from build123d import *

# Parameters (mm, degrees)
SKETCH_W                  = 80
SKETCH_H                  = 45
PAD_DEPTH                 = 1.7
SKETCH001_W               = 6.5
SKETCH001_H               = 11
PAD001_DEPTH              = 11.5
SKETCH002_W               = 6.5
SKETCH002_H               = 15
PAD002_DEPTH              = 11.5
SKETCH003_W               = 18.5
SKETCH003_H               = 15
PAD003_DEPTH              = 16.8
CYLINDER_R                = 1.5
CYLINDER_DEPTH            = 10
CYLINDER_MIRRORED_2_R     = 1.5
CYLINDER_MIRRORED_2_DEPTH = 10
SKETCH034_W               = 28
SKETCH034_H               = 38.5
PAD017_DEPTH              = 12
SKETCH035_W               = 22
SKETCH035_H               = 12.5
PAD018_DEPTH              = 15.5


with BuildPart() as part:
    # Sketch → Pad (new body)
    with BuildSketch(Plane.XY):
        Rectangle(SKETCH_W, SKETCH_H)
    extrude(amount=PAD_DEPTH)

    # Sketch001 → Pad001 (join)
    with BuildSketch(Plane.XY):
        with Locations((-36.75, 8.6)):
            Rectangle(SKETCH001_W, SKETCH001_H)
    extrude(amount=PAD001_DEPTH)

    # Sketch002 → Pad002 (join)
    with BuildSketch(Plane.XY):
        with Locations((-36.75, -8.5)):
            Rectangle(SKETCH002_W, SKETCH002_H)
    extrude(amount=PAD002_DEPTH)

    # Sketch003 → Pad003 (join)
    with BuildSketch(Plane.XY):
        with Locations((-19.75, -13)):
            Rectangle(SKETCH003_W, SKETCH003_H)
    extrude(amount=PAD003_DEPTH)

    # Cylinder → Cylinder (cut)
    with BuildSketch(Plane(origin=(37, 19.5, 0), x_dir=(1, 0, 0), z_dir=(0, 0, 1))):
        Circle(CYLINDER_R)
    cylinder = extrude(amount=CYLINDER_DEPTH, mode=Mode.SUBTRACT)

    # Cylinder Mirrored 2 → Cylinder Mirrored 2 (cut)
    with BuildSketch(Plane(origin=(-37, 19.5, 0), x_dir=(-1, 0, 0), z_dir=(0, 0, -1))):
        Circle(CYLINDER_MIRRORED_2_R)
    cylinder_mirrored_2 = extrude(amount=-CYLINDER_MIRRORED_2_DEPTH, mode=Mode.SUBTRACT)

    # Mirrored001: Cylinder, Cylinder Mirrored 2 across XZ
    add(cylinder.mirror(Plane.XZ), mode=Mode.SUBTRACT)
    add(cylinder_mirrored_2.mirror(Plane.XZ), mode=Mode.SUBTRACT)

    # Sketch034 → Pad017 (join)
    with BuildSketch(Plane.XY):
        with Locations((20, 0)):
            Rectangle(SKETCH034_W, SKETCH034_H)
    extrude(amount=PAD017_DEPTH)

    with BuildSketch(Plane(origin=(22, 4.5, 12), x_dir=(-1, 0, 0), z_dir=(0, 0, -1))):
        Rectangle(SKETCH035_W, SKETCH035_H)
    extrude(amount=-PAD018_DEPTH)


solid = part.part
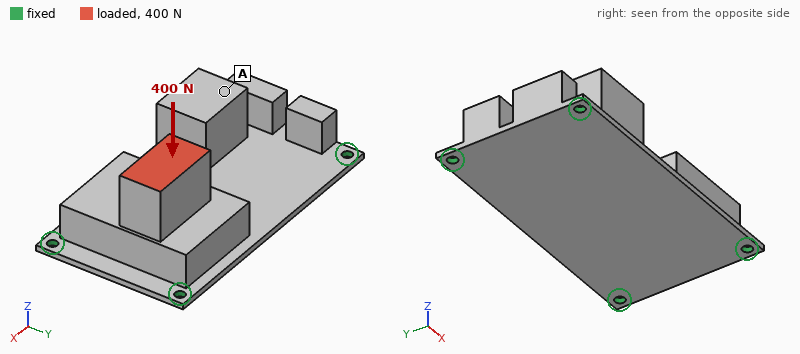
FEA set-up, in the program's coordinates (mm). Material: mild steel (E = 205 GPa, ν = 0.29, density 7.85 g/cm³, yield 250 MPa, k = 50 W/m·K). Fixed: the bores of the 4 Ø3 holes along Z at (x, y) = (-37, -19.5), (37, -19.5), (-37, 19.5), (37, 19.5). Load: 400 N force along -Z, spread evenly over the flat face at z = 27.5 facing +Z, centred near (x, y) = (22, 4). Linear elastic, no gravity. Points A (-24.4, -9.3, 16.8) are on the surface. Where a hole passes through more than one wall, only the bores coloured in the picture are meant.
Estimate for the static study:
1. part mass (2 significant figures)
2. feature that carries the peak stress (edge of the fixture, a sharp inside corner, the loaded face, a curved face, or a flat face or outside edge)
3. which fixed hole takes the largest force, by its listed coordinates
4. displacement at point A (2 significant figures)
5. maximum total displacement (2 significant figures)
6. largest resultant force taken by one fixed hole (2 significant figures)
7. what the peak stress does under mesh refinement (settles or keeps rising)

210 g
edge of the fixture
(37, 19.5)
50 µm
89 µm
230 N
keeps rising
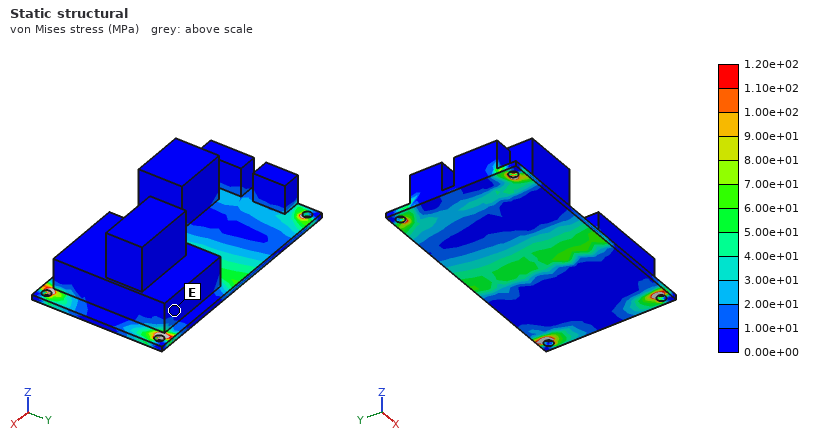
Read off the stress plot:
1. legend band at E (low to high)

0.00e+00 to 1.00e+01 MPa
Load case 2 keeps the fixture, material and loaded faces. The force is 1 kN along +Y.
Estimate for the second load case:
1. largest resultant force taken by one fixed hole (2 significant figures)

980 N
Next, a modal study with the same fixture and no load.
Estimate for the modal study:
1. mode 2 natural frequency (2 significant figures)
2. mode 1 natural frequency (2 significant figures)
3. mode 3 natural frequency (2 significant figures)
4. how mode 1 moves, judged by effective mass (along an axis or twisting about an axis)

2700 Hz
810 Hz
3400 Hz
along Z
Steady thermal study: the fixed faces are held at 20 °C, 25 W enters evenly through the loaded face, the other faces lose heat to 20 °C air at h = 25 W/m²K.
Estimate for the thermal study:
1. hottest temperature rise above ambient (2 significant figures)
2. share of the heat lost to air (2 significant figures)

83 K
37 %
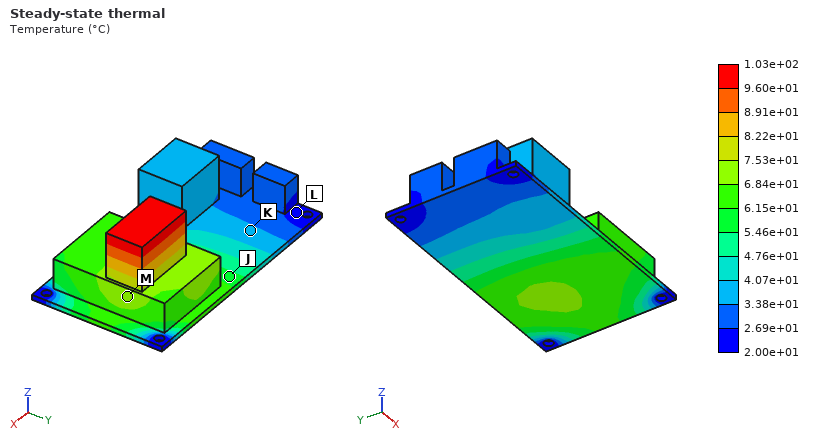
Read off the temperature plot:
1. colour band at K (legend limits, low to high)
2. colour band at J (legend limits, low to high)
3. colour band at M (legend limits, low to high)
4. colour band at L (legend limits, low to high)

3.38e+01 to 4.07e+01 °C
5.46e+01 to 6.15e+01 °C
6.84e+01 to 7.53e+01 °C
2.00e+01 to 2.69e+01 °C
